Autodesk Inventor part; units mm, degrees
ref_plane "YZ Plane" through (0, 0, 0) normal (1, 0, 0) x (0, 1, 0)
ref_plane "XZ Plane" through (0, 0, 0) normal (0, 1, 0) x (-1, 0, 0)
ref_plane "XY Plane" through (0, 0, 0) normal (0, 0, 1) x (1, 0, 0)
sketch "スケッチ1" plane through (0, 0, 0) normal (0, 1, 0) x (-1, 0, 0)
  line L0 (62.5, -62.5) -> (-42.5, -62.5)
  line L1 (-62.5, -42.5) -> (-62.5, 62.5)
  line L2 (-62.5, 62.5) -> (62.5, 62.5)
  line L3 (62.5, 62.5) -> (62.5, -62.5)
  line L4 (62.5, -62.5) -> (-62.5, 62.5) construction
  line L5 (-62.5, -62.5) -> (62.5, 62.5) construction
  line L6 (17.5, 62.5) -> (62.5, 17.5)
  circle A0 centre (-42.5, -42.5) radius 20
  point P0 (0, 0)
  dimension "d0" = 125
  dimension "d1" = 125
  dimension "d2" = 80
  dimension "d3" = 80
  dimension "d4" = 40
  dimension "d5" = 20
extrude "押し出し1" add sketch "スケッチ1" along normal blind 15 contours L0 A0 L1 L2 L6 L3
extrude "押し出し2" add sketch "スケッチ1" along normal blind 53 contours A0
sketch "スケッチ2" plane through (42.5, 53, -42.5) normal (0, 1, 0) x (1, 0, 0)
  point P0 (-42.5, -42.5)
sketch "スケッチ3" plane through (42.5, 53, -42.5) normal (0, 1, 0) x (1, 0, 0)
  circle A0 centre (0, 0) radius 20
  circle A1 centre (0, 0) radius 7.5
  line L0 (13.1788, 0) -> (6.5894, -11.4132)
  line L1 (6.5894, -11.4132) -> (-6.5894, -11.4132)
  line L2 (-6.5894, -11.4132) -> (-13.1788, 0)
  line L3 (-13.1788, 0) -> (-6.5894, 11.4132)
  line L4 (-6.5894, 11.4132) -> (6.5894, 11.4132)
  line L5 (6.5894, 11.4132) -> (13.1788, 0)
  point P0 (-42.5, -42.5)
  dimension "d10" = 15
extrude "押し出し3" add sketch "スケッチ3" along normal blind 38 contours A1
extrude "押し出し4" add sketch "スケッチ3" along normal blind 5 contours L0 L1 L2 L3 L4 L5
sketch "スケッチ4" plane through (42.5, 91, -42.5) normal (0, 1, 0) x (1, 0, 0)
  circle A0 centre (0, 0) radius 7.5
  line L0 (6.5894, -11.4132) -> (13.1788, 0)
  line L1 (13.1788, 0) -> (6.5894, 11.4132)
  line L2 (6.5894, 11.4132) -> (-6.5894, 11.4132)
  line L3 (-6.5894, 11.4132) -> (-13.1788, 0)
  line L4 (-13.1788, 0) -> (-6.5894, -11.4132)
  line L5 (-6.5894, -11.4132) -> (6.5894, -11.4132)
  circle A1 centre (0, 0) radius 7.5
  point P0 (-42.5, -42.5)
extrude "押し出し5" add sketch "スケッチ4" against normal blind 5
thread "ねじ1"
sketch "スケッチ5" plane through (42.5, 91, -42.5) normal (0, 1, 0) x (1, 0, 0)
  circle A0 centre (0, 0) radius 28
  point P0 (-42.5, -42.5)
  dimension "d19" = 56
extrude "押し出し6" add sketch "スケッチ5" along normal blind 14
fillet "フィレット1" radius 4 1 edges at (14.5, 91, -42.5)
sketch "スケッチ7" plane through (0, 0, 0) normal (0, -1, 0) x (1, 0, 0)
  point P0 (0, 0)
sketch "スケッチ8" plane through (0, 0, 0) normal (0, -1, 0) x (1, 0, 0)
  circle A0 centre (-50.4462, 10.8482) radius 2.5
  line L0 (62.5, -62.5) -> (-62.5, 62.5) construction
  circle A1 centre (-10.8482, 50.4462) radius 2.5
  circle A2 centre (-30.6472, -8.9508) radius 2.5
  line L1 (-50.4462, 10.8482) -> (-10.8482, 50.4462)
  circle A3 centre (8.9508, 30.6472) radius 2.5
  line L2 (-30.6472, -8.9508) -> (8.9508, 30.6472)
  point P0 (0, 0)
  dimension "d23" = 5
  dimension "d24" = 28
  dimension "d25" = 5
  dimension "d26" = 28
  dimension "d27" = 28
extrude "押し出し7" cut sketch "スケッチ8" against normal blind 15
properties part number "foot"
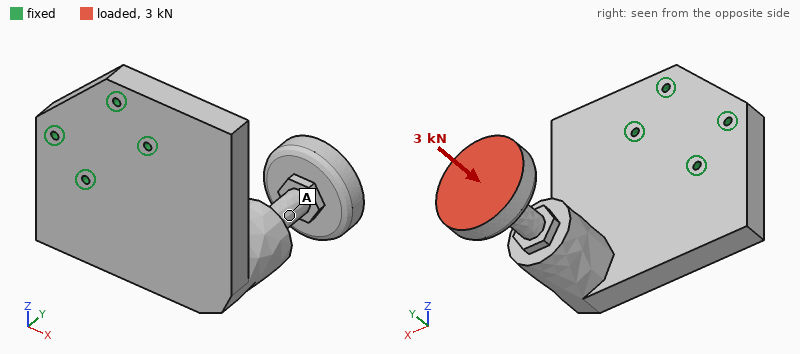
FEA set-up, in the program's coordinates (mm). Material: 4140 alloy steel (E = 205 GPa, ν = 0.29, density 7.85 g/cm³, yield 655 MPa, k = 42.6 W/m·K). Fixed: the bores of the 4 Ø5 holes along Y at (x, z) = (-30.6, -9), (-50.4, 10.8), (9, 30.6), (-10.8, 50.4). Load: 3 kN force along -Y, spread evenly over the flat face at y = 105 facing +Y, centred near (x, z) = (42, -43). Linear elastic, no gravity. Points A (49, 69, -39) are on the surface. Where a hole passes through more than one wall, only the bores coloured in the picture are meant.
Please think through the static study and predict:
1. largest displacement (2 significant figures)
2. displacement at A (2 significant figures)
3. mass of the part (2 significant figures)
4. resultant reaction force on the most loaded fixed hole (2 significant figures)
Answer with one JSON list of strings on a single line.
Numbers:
["0.19 mm", "0.12 mm", "2.4 kg", "3.5 kN"]
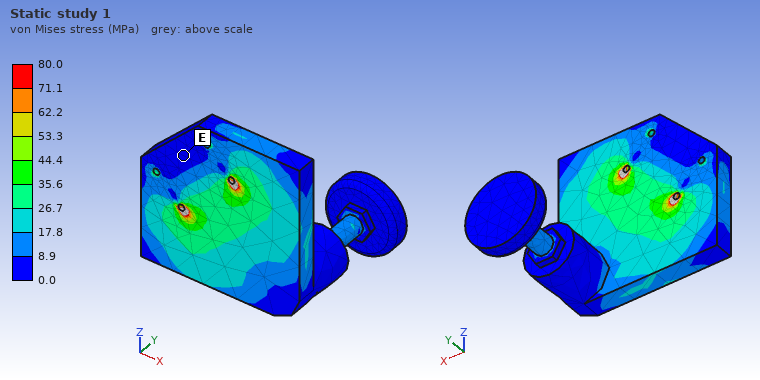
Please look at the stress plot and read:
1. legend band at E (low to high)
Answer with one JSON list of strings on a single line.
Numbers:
["0.0 to 8.9 MPa"]
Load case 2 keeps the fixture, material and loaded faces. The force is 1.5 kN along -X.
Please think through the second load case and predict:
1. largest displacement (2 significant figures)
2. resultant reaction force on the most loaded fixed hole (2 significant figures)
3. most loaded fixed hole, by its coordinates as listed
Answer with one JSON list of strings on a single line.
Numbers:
["0.32 mm", "3.0 kN", "(9, 30.6)"]
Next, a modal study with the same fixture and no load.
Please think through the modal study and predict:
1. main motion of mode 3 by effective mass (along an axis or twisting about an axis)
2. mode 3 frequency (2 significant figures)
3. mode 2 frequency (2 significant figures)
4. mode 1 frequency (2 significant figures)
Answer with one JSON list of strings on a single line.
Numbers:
["along Y", "1400 Hz", "830 Hz", "610 Hz"]
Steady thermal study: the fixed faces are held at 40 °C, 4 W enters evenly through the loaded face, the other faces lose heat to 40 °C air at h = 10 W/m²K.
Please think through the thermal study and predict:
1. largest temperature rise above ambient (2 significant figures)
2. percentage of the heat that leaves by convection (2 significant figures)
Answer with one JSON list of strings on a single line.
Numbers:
["20 K", "43 %"]
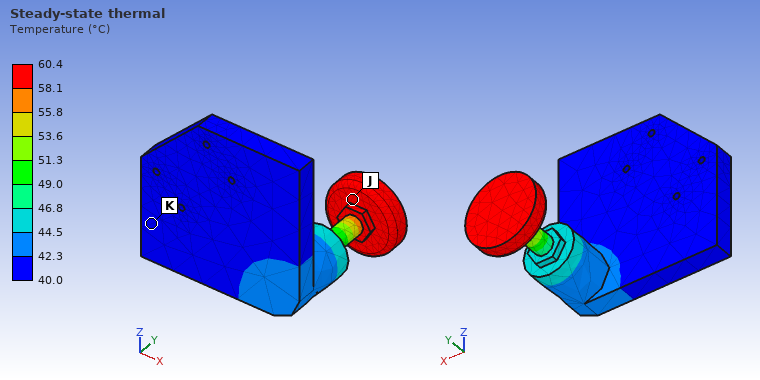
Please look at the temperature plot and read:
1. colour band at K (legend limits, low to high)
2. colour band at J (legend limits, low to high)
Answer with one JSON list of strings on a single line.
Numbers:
["40.0 to 42.3 °C", "58.1 to 60.4 °C"]
